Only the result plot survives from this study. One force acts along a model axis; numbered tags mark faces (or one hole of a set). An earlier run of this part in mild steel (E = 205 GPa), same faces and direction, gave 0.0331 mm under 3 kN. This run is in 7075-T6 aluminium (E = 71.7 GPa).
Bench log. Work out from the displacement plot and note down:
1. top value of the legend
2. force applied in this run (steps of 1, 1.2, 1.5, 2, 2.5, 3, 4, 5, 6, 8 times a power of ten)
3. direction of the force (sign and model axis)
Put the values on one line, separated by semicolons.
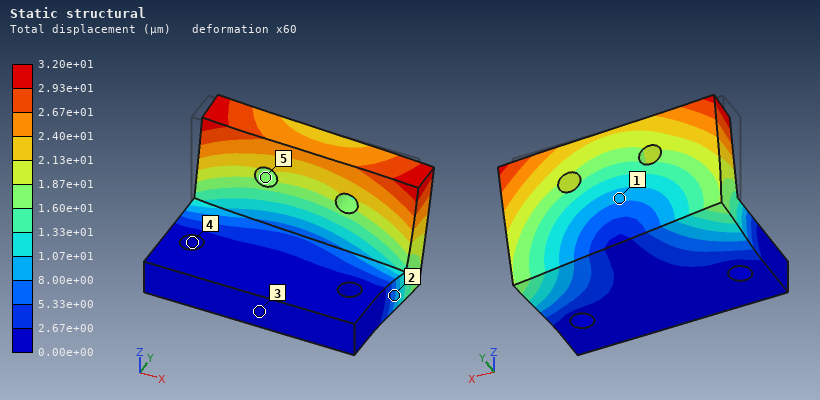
3.20e+01 µm; 1 kN; +X
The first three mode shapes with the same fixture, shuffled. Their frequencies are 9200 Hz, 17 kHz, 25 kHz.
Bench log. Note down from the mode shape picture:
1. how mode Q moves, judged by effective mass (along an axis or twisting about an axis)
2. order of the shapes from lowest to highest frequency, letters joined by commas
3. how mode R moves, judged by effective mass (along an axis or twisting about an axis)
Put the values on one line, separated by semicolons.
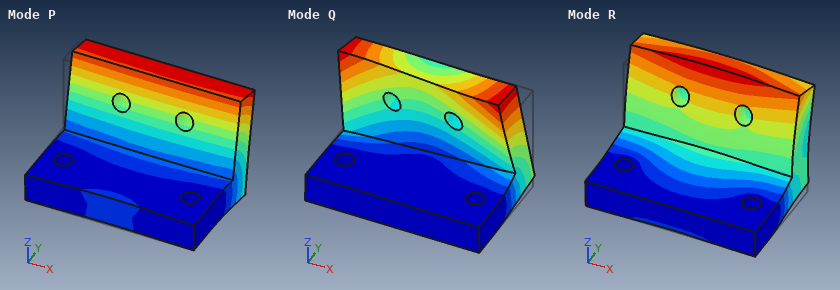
along X; P, Q, R; along Z
